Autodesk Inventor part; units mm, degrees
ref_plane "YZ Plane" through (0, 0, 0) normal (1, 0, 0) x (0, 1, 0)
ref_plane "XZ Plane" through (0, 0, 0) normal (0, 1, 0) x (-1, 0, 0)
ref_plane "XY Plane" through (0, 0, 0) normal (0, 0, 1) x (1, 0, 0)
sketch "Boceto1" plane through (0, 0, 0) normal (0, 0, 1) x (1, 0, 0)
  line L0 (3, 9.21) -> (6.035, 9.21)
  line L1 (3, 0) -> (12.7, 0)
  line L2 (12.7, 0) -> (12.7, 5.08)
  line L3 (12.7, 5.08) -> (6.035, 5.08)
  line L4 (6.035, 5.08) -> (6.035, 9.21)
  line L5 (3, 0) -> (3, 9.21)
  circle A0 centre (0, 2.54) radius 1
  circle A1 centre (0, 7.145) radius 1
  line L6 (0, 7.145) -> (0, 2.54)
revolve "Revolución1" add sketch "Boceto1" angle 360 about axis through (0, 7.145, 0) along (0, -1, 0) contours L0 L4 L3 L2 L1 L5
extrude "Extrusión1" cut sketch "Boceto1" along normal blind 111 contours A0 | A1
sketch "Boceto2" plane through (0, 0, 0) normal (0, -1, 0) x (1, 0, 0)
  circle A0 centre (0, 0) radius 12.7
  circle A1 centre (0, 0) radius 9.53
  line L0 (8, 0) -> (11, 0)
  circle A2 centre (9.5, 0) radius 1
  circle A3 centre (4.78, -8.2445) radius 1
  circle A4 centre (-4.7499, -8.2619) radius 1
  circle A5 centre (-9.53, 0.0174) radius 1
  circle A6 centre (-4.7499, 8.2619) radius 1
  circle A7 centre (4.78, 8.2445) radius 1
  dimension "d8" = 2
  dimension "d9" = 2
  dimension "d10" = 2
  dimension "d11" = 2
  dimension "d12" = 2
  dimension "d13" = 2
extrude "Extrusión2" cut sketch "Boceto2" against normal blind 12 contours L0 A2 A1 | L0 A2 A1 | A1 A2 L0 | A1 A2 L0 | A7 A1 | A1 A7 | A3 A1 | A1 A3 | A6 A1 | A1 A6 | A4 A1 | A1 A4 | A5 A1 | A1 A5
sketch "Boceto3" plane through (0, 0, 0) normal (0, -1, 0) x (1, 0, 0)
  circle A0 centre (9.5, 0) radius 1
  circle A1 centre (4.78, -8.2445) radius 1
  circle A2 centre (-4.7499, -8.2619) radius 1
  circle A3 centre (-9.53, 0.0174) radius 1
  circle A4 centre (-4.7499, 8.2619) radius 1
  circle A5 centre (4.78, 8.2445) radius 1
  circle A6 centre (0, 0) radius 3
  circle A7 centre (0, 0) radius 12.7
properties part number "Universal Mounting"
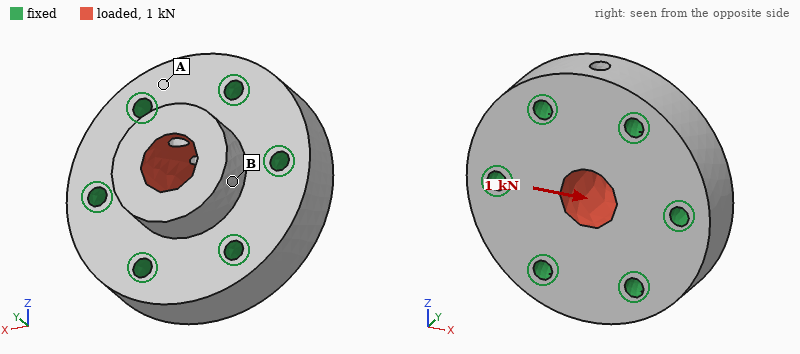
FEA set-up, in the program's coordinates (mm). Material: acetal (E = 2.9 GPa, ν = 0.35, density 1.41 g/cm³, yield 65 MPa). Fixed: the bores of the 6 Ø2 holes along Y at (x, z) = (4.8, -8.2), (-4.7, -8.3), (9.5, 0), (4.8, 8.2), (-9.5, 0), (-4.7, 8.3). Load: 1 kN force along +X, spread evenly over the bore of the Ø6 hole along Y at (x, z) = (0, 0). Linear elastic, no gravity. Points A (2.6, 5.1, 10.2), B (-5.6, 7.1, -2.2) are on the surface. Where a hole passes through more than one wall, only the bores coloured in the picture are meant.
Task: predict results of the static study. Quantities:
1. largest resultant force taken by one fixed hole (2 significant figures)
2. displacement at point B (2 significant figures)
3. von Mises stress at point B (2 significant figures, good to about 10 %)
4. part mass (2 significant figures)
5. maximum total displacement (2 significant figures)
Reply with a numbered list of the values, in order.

1. 270 N
2. 37 µm
3. 4.5 MPa
4. 3.7 g
5. 55 µm
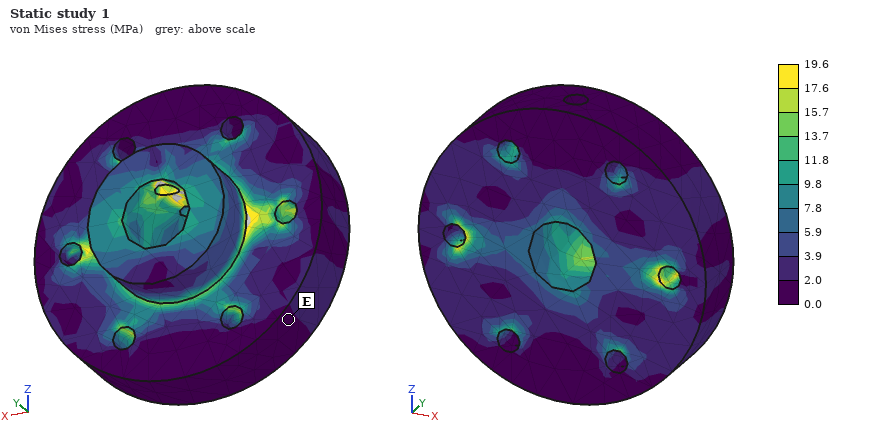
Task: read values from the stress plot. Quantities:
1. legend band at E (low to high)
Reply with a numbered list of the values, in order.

1. 0.0 to 2.0 MPa
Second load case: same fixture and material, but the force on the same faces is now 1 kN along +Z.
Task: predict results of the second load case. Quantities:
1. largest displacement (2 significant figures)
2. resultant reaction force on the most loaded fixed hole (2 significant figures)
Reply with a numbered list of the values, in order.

1. 53 µm
2. 240 N
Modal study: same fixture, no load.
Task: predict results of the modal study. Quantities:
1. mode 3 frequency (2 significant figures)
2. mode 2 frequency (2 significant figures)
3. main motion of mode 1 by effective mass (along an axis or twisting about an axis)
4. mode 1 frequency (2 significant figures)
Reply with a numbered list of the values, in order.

1. 26 kHz
2. 25 kHz
3. along Y
4. 23 kHz
